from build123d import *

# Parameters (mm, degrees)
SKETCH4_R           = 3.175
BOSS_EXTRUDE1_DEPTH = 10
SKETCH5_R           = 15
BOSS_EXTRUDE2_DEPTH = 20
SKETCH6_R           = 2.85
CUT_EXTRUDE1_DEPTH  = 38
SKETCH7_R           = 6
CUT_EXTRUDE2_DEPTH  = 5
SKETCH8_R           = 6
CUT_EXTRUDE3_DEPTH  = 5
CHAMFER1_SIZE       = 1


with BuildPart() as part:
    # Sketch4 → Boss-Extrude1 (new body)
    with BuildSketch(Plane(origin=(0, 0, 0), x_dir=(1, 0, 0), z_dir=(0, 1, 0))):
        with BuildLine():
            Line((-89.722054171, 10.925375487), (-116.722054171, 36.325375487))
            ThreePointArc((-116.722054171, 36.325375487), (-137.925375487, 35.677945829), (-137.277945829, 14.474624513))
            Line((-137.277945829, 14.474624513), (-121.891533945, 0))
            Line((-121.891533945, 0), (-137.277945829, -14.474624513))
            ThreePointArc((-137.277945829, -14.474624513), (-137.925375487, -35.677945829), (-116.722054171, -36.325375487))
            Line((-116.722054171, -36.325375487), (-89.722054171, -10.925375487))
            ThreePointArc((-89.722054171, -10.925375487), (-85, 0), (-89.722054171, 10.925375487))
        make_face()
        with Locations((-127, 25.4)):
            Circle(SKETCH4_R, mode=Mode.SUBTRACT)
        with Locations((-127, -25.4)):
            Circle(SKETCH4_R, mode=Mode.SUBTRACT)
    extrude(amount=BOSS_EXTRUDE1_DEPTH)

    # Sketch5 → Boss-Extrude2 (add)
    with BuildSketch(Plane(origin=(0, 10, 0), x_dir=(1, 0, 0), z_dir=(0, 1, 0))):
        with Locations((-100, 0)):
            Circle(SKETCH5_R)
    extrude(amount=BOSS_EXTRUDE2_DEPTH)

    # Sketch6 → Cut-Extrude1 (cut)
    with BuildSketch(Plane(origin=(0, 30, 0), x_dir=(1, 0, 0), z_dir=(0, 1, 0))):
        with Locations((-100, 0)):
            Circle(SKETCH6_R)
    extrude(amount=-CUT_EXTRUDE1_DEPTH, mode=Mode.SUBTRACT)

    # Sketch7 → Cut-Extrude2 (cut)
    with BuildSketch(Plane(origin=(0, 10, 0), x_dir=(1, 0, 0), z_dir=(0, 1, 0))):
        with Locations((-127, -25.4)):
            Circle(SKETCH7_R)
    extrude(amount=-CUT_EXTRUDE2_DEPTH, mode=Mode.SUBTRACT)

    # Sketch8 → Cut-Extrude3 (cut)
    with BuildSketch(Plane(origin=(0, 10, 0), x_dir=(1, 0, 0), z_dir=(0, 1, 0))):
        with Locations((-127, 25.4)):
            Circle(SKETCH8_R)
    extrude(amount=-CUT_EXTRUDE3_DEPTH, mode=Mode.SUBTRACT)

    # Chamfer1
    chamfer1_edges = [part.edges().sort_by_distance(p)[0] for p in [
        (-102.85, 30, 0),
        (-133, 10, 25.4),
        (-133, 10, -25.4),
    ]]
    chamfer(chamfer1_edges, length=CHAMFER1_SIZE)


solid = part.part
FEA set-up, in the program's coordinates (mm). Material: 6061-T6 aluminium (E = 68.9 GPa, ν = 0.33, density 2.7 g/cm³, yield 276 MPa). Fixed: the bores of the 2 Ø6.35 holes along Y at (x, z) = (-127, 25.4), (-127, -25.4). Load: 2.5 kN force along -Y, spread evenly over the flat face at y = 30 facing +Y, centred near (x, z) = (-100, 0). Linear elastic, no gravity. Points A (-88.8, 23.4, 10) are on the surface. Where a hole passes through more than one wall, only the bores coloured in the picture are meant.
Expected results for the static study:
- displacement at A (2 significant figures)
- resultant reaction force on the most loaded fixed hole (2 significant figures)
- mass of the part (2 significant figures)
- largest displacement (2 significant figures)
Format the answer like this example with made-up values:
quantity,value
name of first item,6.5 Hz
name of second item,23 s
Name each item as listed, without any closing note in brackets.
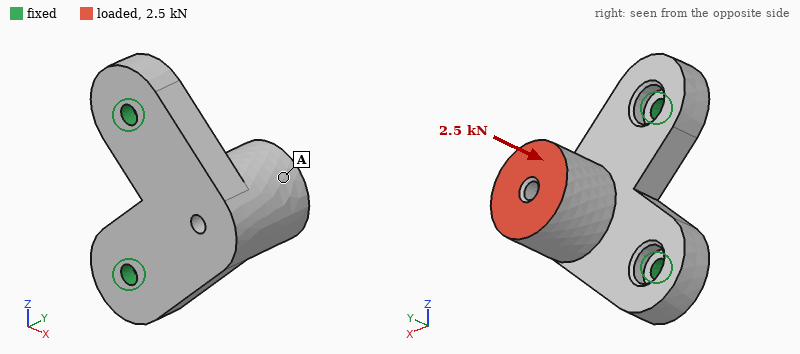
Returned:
quantity,value
displacement at A,0.25 mm
resultant reaction force on the most loaded fixed hole,1.3 kN
mass of the part,110 g
largest displacement,0.29 mm
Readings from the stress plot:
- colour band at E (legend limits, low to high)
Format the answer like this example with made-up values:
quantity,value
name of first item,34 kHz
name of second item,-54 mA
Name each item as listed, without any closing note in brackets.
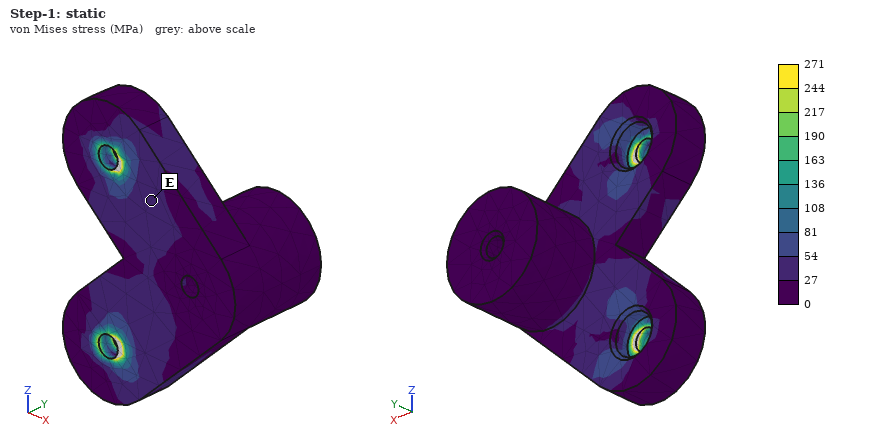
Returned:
quantity,value
colour band at E,27 to 54 MPa
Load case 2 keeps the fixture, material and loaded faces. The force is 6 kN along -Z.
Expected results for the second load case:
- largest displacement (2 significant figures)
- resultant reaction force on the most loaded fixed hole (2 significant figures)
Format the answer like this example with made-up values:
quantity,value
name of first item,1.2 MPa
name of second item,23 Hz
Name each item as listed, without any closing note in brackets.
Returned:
quantity,value
largest displacement,0.14 mm
resultant reaction force on the most loaded fixed hole,5.4 kN
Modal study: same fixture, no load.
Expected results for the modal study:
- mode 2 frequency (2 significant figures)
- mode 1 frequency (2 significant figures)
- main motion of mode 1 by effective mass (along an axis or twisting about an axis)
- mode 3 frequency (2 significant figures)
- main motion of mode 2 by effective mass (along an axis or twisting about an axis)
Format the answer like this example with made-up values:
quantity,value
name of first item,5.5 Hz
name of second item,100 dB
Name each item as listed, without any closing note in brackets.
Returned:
quantity,value
mode 2 frequency,7500 Hz
mode 1 frequency,2200 Hz
main motion of mode 1 by effective mass,along Y
mode 3 frequency,9300 Hz
main motion of mode 2 by effective mass,along Z
